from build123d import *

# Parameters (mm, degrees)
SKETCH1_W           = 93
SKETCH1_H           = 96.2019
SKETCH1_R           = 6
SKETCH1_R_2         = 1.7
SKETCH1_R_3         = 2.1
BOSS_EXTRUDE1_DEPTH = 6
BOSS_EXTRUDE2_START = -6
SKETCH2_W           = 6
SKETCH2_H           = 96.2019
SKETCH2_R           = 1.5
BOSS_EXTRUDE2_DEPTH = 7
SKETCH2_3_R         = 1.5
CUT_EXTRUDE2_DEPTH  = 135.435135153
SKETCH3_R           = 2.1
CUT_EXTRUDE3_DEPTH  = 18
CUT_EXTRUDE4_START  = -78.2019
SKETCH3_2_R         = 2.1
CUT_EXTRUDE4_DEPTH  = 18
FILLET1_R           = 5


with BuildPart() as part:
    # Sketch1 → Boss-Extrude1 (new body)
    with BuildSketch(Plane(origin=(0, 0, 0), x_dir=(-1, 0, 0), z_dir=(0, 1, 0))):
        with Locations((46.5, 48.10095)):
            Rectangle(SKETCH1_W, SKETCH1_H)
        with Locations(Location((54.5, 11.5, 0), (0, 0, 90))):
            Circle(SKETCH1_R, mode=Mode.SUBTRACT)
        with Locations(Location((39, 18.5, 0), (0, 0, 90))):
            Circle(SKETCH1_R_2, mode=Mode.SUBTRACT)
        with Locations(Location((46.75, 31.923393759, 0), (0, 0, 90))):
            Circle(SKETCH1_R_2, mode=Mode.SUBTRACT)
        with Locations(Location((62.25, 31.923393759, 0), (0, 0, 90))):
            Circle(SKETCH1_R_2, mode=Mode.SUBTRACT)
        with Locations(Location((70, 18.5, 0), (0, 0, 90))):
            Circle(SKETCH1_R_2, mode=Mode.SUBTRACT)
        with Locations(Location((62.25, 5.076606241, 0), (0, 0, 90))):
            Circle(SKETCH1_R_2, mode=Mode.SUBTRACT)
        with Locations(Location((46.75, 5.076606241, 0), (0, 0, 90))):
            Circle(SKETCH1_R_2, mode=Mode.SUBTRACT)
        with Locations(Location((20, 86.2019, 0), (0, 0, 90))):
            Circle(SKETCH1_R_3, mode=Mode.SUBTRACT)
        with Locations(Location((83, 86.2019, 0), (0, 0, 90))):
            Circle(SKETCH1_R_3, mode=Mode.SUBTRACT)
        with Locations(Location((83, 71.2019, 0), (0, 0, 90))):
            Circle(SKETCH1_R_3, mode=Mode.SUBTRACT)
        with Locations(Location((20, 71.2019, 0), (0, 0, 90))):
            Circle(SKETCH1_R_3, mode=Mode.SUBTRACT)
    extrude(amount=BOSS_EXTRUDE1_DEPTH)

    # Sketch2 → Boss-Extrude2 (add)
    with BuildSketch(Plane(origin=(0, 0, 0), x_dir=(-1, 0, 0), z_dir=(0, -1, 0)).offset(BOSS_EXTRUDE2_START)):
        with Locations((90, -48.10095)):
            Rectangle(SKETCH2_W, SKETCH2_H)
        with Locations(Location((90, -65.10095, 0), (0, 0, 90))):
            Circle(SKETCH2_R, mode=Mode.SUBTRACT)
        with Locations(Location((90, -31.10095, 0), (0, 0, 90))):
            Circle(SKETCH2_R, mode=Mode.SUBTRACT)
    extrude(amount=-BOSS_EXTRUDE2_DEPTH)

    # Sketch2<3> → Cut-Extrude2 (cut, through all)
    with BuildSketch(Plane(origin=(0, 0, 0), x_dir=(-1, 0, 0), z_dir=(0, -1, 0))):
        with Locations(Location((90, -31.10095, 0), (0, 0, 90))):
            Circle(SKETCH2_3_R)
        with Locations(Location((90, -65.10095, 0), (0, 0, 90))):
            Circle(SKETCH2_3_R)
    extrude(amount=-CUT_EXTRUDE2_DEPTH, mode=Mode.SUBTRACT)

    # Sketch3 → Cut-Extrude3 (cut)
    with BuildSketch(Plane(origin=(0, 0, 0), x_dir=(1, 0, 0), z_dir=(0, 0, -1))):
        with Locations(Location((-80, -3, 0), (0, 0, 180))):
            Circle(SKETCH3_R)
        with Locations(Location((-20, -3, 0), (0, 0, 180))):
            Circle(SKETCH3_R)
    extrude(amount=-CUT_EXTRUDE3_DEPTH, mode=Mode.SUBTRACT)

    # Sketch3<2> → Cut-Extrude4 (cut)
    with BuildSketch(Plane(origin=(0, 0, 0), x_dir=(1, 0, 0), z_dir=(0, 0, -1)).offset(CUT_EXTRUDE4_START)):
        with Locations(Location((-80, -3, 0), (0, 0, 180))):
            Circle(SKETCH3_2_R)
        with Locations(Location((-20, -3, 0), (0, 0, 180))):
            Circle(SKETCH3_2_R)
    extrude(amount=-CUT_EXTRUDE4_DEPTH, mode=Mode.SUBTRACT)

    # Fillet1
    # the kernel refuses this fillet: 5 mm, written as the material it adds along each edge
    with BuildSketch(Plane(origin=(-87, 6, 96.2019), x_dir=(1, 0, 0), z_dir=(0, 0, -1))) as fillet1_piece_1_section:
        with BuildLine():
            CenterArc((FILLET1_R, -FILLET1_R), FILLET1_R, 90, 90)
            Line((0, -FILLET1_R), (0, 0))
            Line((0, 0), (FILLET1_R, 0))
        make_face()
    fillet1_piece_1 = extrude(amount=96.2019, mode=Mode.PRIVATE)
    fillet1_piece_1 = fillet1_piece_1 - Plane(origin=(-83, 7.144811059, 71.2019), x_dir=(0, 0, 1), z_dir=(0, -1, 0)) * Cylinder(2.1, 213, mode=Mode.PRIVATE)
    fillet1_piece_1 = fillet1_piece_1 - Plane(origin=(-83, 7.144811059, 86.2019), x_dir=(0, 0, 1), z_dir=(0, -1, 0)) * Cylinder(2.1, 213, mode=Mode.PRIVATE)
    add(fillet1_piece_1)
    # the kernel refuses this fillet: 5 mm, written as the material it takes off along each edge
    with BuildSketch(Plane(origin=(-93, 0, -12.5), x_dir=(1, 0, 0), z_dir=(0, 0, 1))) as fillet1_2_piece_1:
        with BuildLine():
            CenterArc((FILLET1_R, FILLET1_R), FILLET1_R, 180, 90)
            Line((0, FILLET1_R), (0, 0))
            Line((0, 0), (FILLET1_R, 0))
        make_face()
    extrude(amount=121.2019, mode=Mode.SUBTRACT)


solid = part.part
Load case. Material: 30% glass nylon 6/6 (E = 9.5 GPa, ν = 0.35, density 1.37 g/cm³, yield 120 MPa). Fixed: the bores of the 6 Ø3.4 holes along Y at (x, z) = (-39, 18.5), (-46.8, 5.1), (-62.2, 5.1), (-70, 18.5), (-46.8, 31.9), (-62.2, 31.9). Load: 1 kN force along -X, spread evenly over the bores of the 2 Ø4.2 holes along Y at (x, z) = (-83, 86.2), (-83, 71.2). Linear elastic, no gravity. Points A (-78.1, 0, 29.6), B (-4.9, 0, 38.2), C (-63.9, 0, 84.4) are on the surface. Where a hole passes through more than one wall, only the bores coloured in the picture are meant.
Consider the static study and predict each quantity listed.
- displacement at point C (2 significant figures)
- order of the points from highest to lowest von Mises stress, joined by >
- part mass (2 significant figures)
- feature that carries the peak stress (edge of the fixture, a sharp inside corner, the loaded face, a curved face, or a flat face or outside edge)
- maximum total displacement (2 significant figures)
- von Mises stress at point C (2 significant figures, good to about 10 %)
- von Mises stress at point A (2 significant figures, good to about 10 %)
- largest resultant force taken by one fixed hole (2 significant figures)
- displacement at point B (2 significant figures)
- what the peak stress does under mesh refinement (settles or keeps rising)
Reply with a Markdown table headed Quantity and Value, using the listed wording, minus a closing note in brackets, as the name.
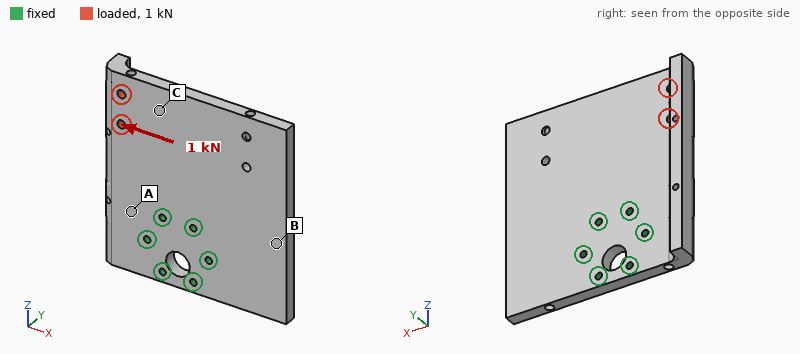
| Quantity | Value |
|---|---|
| displacement at point C | 0.11 mm |
| order of the points from highest to lowest von Mises stress, joined by > | A > C > B |
| part mass | 76 g |
| feature that carries the peak stress | edge of the fixture |
| maximum total displacement | 0.15 mm |
| von Mises stress at point C | 3.4 MPa |
| von Mises stress at point A | 6.8 MPa |
| largest resultant force taken by one fixed hole | 950 N |
| displacement at point B | 0.060 mm |
| what the peak stress does under mesh refinement | keeps rising |
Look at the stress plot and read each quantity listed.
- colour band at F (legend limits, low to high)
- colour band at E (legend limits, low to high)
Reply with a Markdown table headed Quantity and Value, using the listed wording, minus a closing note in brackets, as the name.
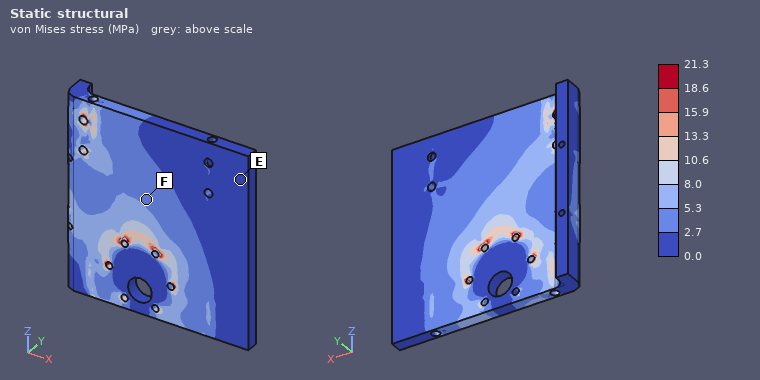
| Quantity | Value |
|---|---|
| colour band at F | 2.7 to 5.3 MPa |
| colour band at E | 0.0 to 2.7 MPa |
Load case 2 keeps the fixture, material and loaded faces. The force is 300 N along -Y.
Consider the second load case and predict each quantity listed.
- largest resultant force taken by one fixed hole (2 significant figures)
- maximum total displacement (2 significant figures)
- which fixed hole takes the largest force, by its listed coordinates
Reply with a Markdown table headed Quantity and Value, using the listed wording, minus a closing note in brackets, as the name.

| Quantity | Value |
|---|---|
| largest resultant force taken by one fixed hole | 610 N |
| maximum total displacement | 1.5 mm |
| which fixed hole takes the largest force, by its listed coordinates | (-62.2, 31.9) |
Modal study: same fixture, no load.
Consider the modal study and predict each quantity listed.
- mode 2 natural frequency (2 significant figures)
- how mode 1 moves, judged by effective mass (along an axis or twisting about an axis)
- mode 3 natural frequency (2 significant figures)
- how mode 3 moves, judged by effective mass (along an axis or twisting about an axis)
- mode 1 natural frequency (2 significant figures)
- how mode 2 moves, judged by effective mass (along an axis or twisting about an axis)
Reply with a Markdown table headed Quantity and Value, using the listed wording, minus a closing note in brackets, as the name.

| Quantity | Value |
|---|---|
| mode 2 natural frequency | 810 Hz |
| how mode 1 moves, judged by effective mass | along Y |
| mode 3 natural frequency | 1600 Hz |
| how mode 3 moves, judged by effective mass | along Y |
| mode 1 natural frequency | 580 Hz |
| how mode 2 moves, judged by effective mass | twisting about Z |
